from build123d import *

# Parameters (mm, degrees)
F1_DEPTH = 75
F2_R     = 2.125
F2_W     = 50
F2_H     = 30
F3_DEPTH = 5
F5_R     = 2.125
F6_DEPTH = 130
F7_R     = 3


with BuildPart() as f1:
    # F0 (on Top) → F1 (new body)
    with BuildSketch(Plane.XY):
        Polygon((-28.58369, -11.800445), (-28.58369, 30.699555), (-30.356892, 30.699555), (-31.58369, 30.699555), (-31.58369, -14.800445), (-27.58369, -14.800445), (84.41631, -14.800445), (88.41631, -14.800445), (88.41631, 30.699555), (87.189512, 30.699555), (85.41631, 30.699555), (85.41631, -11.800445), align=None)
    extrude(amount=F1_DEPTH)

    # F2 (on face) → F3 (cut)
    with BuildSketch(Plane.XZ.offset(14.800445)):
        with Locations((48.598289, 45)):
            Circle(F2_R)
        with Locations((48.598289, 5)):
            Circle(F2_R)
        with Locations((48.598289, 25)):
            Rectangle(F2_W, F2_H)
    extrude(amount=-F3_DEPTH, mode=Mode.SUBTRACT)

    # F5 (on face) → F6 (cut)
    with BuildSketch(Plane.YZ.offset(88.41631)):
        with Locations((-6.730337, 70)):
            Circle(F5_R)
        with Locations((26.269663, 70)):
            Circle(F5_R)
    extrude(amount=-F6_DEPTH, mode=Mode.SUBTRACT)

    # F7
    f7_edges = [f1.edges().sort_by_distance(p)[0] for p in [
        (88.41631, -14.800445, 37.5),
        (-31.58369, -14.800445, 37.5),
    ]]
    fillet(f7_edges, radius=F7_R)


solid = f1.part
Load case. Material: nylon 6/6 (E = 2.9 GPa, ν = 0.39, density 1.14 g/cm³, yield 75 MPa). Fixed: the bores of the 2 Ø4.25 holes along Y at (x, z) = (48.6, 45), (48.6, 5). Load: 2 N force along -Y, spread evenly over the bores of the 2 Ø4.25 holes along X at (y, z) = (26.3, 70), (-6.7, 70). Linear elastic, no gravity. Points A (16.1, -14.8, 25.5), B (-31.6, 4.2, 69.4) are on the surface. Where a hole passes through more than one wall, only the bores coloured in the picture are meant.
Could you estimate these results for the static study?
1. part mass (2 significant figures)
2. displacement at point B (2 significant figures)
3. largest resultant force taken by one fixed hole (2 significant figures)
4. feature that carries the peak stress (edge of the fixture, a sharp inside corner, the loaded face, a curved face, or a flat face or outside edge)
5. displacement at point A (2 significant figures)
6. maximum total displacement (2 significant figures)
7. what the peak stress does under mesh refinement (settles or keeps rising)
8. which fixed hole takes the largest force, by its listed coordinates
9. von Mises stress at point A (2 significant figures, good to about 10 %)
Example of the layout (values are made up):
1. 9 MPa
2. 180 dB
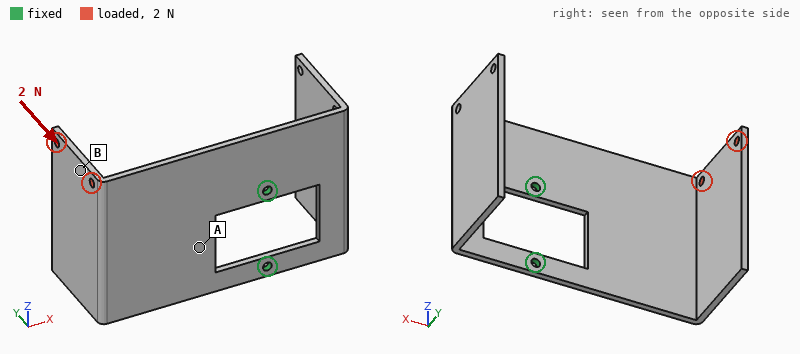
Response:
1. 47 g
2. 1.4 mm
3. 2.3 N
4. edge of the fixture
5. 0.25 mm
6. 1.6 mm
7. keeps rising
8. (48.6, 45)
9. 0.57 MPa
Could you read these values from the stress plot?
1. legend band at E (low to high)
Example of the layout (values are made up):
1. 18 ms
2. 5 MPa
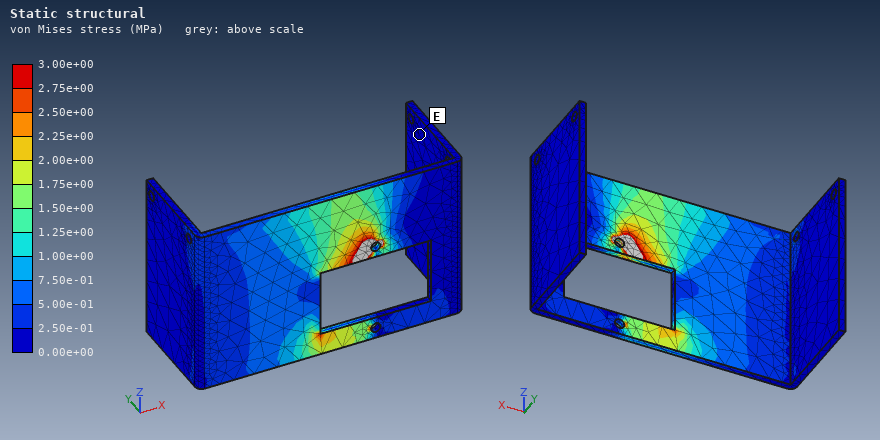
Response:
1. 0.00e+00 to 2.50e-01 MPa
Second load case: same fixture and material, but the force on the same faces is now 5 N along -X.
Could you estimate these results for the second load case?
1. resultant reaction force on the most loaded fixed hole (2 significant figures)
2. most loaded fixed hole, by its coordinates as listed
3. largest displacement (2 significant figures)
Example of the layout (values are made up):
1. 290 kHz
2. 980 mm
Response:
1. 7.4 N
2. (48.6, 45)
3. 1.8 mm
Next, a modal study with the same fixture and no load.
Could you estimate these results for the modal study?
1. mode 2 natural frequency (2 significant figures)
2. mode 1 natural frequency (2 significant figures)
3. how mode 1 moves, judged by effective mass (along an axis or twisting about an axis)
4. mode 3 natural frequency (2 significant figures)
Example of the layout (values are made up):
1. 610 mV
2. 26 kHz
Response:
1. 110 Hz
2. 50 Hz
3. along Y
4. 130 Hz
